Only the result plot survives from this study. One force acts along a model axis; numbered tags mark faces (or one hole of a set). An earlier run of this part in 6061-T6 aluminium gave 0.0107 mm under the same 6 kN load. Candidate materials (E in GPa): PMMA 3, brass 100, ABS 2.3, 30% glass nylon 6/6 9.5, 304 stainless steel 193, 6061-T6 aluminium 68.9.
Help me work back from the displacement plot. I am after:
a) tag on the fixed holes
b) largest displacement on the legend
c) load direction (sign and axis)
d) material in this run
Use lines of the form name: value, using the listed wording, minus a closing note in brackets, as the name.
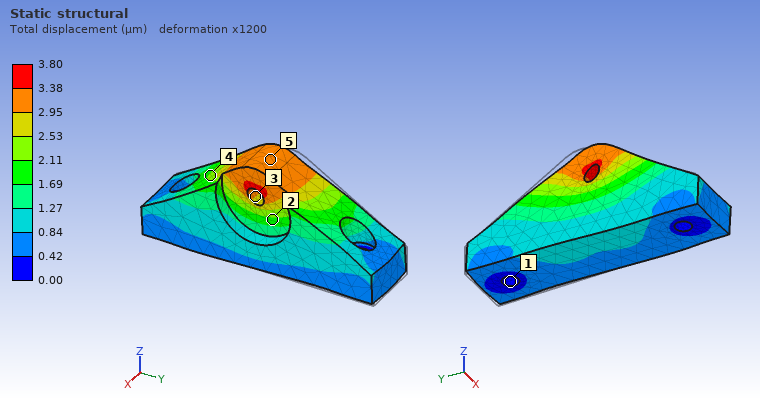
tag on the fixed holes: 1
largest displacement on the legend: 3.80 µm
load direction: -Y
material in this run: 304 stainless steel
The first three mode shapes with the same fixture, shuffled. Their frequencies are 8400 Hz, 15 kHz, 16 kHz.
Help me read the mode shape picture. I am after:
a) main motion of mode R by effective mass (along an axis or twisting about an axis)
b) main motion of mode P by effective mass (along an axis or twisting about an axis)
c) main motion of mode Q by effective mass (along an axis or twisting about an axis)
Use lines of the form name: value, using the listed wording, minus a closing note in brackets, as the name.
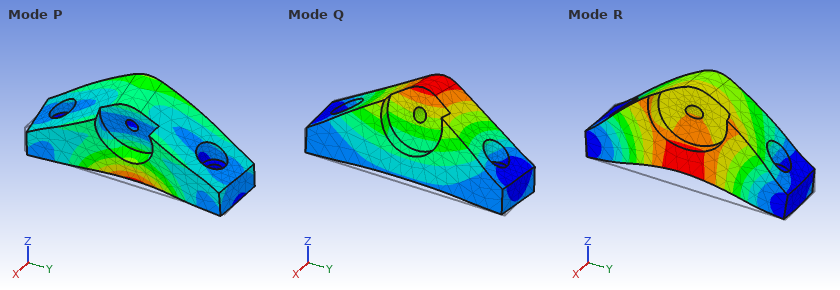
main motion of mode R by effective mass: along Z
main motion of mode P by effective mass: along X
main motion of mode Q by effective mass: along X
